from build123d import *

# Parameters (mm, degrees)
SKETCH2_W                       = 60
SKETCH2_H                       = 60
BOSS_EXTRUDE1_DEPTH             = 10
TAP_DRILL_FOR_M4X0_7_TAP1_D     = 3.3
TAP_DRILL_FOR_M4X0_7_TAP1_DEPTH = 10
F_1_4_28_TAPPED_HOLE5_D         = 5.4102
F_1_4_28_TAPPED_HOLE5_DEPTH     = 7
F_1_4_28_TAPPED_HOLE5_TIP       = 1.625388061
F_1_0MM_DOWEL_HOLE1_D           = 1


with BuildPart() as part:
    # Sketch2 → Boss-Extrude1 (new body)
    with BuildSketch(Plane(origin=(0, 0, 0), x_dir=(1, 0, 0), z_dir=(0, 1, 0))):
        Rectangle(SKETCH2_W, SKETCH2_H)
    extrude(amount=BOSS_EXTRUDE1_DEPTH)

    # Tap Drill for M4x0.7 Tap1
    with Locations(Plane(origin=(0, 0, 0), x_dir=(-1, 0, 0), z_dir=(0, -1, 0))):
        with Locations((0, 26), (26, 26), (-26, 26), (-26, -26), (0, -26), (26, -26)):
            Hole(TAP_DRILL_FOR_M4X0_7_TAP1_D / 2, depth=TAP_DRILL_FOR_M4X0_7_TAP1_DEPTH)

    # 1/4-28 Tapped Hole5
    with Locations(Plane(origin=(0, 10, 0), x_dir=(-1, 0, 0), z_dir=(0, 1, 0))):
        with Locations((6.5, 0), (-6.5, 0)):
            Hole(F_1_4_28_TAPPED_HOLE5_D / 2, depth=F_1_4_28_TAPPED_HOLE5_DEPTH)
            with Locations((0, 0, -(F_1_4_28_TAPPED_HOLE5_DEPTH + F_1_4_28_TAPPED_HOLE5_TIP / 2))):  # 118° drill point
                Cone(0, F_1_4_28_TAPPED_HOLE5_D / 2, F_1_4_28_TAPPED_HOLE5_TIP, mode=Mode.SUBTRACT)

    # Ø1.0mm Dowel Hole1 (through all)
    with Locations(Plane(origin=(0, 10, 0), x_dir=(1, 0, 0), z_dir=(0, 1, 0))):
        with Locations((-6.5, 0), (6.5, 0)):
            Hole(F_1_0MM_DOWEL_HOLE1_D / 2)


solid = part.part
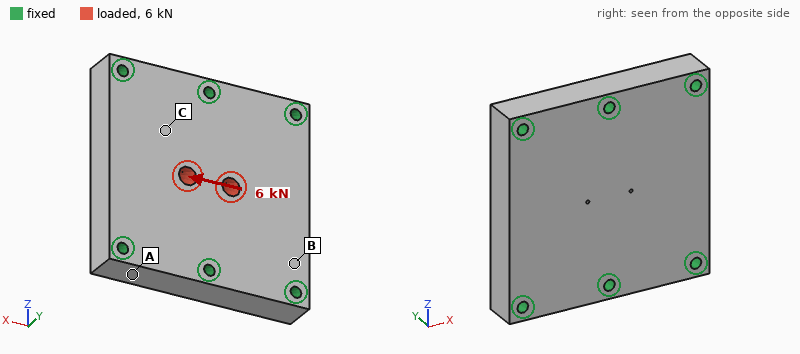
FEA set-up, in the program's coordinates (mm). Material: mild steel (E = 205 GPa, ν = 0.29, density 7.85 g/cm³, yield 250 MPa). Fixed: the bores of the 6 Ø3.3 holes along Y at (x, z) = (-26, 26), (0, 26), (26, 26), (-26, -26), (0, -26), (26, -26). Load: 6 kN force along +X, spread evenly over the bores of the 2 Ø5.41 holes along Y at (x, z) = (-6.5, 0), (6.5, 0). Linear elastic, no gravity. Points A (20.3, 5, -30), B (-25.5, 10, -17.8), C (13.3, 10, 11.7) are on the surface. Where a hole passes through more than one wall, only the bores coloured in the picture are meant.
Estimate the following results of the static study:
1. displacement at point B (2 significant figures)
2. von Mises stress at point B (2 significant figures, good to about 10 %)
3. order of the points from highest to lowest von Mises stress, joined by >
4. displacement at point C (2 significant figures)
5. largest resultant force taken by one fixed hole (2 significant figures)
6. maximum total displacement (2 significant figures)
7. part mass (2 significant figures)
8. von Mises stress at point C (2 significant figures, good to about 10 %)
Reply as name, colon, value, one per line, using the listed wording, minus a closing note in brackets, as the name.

displacement at point B: 0.68 µm
von Mises stress at point B: 7.4 MPa
order of the points from highest to lowest von Mises stress, joined by >: C > B > A
displacement at point C: 1.2 µm
largest resultant force taken by one fixed hole: 1.3 kN
maximum total displacement: 3.1 µm
part mass: 280 g
von Mises stress at point C: 13 MPa
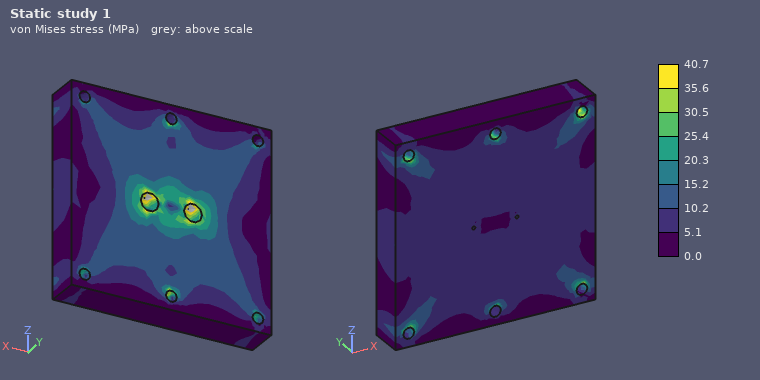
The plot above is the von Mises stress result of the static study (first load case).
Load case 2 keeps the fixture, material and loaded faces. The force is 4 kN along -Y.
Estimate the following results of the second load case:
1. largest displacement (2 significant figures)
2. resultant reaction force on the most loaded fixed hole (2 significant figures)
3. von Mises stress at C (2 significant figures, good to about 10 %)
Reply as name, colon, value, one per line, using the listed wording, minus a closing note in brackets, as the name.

largest displacement: 8.0 µm
resultant reaction force on the most loaded fixed hole: 1.3 kN
von Mises stress at C: 14 MPa
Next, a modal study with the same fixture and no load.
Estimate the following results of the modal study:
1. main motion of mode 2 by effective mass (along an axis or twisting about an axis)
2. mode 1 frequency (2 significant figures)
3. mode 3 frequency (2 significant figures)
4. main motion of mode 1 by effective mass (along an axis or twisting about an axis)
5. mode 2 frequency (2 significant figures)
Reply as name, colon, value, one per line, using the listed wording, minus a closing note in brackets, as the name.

main motion of mode 2 by effective mass: twisting about Z
mode 1 frequency: 14 kHz
mode 3 frequency: 25 kHz
main motion of mode 1 by effective mass: along Y
mode 2 frequency: 17 kHz
